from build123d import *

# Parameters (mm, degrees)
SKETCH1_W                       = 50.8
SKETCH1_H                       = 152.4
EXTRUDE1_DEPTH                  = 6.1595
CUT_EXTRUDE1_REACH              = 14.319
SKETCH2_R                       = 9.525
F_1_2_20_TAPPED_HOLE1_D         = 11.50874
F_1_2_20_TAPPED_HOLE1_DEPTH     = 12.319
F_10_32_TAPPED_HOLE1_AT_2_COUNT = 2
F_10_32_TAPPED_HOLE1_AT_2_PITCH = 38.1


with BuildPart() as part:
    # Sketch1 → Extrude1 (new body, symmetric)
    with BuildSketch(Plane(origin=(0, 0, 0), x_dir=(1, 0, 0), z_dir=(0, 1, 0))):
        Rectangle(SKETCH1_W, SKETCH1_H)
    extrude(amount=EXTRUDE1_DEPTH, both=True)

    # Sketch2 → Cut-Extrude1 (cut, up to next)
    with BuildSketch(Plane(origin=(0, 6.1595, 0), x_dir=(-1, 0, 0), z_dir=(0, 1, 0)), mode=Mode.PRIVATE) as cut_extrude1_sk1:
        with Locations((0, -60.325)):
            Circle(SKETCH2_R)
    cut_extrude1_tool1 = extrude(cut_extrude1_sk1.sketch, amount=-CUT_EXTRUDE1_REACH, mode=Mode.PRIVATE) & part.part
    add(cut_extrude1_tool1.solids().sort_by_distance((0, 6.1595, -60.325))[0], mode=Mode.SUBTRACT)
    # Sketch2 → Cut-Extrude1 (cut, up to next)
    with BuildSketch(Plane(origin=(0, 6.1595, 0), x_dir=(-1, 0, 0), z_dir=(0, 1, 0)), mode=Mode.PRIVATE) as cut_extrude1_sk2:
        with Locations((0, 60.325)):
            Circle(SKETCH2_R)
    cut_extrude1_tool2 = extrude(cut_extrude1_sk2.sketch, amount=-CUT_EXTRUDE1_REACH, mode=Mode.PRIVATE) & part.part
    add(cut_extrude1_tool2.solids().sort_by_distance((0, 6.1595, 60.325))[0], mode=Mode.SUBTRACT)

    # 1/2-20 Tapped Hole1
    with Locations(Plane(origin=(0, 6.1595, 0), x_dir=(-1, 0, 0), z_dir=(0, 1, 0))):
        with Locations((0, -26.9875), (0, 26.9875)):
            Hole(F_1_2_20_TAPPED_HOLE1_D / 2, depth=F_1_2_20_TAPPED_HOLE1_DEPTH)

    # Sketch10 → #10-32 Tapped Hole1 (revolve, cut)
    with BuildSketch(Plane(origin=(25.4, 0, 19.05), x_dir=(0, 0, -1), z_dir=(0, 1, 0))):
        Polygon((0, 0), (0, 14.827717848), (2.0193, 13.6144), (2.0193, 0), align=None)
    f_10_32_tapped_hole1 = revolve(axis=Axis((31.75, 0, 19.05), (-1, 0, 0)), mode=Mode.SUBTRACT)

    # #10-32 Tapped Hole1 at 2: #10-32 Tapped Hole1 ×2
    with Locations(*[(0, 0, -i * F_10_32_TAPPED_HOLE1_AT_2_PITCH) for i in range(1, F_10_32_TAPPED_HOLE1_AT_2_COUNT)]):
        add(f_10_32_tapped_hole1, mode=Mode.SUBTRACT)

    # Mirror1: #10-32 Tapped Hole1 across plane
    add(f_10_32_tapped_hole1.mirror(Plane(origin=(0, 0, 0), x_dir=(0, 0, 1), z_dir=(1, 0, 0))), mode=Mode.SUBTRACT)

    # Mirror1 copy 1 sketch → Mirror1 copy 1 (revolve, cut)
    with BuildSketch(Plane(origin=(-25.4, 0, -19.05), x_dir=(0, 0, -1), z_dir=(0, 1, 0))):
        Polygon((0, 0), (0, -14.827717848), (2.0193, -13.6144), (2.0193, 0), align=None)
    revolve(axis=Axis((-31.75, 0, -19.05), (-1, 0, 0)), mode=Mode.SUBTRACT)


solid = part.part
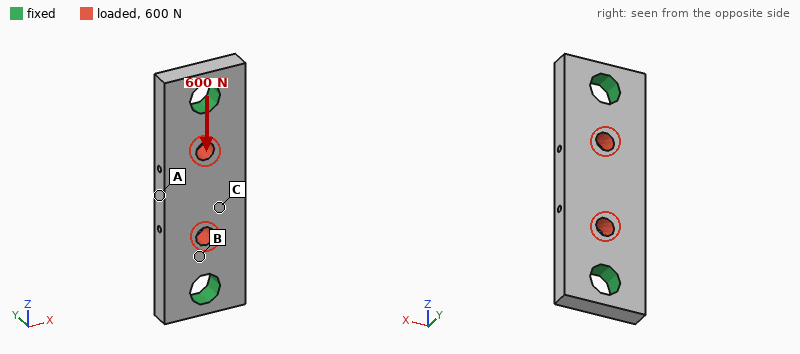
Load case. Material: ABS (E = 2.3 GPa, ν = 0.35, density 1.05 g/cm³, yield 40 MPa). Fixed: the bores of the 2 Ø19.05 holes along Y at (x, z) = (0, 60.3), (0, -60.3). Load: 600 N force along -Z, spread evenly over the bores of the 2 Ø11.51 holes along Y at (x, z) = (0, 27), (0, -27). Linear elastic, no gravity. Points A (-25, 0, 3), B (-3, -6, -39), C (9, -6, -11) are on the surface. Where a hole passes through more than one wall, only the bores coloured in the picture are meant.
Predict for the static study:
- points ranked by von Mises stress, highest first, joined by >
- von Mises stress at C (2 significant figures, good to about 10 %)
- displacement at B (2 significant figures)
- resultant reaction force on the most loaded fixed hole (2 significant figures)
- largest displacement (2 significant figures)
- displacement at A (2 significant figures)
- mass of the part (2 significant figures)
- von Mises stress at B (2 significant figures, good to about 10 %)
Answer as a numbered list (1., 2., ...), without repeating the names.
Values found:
1. B > C > A
2. 0.28 MPa
3. 4.6 µm
4. 300 N
5. 12 µm
6. 7.3 µm
7. 89 g
8. 0.87 MPa
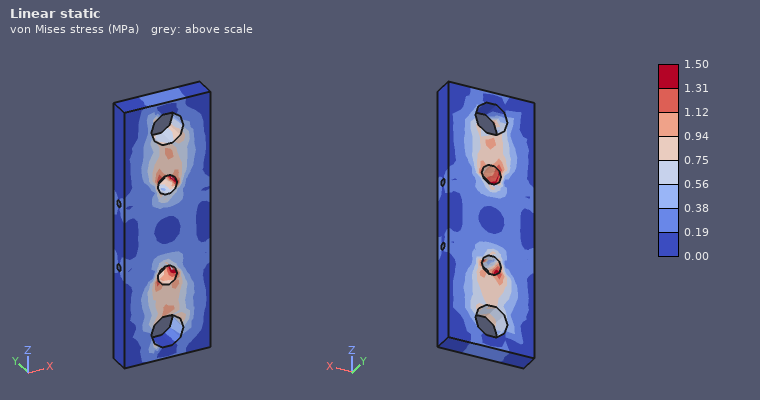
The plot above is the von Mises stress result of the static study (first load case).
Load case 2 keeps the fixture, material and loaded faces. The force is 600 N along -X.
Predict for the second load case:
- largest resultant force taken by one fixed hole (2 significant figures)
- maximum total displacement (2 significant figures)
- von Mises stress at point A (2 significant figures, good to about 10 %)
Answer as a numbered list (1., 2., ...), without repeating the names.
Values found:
1. 300 N
2. 39 µm
3. 0.85 MPa
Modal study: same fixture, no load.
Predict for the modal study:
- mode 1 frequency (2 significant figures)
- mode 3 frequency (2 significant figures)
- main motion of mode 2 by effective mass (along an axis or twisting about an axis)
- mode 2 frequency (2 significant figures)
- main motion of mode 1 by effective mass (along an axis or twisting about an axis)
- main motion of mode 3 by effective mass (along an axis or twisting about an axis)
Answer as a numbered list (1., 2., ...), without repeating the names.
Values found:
1. 1500 Hz
2. 2700 Hz
3. twisting about Z
4. 1900 Hz
5. along Y
6. along X
